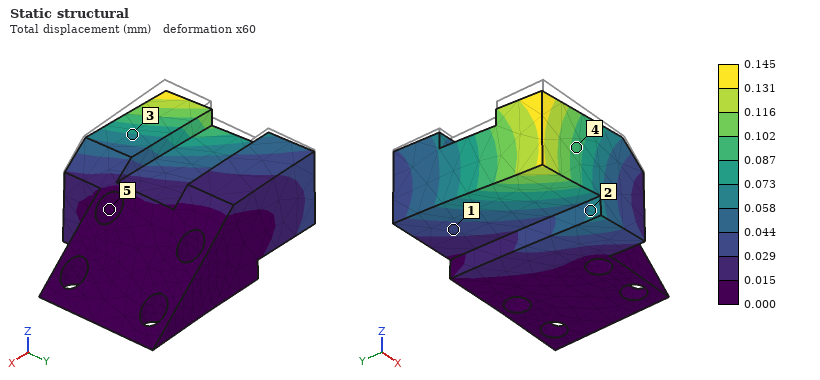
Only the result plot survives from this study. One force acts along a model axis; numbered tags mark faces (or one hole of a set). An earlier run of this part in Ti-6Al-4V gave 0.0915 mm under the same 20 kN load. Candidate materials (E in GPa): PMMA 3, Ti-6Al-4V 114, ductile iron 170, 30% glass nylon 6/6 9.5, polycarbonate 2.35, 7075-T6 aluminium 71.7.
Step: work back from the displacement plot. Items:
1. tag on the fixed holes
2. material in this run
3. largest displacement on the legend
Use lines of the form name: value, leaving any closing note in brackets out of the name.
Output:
tag on the fixed holes: 5
material in this run: 7075-T6 aluminium
largest displacement on the legend: 0.145 mm
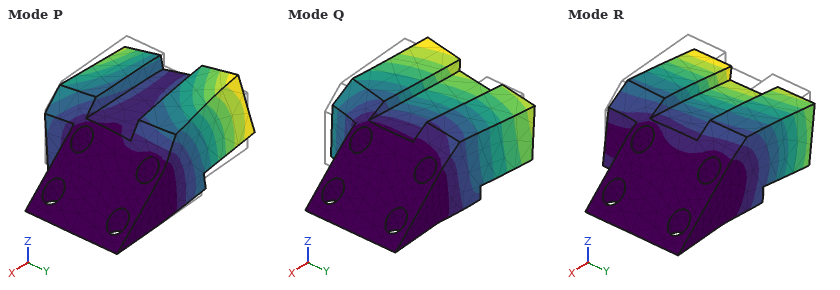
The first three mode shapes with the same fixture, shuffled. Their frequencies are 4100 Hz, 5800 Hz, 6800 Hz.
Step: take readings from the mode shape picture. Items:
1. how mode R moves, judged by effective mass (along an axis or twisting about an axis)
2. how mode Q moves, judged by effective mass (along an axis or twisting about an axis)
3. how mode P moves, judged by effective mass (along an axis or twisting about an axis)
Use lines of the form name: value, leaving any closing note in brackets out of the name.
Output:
how mode R moves, judged by effective mass: along Z
how mode Q moves, judged by effective mass: along Y
how mode P moves, judged by effective mass: twisting about X
